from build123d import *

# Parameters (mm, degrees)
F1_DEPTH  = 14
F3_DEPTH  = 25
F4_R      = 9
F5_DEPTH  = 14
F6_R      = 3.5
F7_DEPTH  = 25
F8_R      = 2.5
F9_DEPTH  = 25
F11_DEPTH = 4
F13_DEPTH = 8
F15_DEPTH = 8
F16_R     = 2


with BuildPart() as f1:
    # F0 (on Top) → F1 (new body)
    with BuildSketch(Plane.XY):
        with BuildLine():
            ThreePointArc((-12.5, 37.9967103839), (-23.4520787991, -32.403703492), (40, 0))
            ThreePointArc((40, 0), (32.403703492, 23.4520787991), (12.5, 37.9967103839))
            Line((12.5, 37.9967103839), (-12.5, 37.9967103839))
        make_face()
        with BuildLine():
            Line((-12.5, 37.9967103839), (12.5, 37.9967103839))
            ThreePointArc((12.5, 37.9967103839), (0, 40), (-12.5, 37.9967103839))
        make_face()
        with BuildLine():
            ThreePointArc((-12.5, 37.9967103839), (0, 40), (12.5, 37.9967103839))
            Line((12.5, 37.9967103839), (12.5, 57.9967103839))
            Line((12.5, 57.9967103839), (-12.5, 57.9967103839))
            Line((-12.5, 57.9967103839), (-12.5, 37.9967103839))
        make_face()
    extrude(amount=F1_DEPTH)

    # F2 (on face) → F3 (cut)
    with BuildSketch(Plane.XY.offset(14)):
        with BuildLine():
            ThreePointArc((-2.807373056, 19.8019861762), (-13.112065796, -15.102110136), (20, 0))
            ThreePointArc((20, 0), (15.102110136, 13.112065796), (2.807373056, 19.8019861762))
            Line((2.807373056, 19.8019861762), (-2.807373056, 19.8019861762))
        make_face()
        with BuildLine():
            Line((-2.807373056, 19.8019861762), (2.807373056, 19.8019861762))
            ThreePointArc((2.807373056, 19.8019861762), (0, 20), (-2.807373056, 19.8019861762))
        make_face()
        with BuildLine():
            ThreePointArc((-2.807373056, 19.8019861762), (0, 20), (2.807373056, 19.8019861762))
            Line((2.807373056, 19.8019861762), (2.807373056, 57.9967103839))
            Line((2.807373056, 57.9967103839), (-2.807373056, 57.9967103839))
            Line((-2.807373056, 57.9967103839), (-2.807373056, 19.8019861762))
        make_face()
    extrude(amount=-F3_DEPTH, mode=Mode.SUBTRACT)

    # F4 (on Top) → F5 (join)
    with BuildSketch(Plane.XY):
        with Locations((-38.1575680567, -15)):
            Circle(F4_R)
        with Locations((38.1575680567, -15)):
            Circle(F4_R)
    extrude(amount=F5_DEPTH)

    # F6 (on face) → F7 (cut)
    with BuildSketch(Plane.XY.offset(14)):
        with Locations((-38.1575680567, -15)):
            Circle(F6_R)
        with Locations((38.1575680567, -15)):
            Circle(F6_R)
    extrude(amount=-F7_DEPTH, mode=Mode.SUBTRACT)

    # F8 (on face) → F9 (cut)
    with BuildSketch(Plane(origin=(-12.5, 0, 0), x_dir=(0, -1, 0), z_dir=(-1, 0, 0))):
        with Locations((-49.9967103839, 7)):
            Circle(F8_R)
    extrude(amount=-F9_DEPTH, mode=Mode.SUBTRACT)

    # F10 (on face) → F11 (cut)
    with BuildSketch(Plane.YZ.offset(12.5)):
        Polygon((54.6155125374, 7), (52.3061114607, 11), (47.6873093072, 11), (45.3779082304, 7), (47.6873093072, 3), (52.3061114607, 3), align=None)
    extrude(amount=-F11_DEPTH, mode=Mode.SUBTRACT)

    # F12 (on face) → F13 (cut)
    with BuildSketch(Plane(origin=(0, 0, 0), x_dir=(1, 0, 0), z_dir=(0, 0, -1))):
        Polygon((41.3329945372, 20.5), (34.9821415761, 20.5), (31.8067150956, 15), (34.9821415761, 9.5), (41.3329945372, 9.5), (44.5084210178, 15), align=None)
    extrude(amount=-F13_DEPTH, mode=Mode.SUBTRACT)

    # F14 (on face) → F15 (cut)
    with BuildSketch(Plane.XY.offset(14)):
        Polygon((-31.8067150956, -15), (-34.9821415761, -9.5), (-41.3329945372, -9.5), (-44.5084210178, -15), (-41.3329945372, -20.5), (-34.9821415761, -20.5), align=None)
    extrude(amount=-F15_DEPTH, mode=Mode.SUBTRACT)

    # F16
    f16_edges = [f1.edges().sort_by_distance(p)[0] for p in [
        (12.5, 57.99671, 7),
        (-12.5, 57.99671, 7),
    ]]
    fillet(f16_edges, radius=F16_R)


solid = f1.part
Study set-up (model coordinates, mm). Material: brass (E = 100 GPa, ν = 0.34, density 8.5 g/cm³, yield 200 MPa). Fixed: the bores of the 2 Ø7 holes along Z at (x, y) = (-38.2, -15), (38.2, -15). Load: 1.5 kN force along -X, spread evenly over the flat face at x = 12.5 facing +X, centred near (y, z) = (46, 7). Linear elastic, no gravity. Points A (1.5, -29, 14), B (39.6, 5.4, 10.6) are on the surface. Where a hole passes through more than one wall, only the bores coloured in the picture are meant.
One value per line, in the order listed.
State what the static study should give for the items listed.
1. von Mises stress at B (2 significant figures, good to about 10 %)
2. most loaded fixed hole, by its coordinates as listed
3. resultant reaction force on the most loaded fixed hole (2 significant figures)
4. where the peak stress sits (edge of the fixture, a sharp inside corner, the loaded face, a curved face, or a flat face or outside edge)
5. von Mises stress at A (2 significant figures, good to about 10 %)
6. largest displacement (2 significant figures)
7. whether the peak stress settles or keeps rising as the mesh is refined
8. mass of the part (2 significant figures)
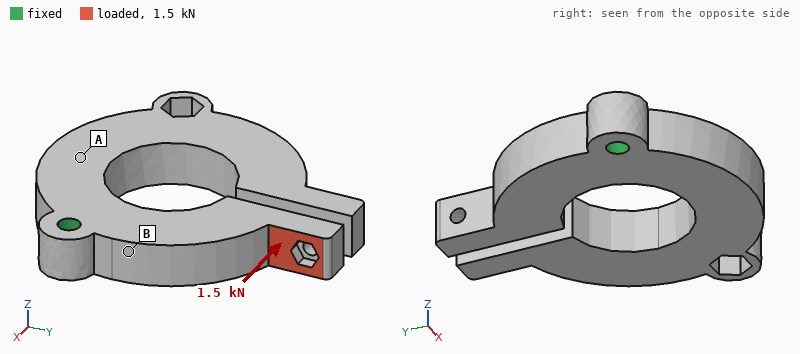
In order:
55 MPa
(38.2, -15)
3.0 kN
edge of the fixture
14 MPa
0.27 mm
keeps rising
490 g
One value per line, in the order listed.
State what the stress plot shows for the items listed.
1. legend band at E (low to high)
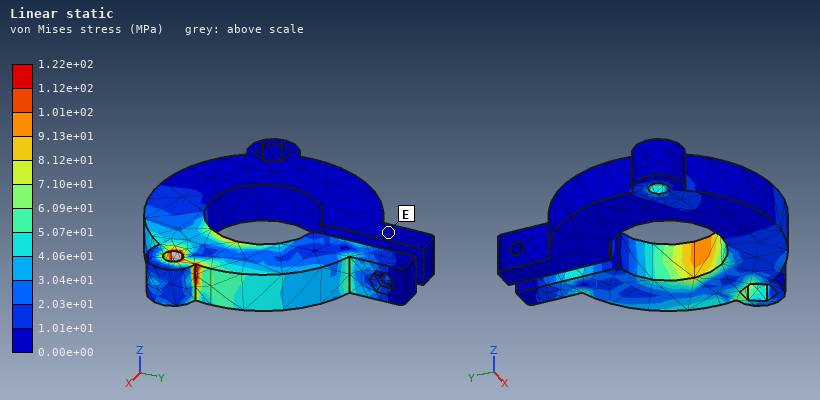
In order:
0.00e+00 to 1.01e+01 MPa
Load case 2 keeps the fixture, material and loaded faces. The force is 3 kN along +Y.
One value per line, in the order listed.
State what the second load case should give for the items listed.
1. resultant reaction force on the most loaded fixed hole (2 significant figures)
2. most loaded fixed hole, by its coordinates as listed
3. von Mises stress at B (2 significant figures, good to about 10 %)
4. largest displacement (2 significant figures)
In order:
2.5 kN
(38.2, -15)
34 MPa
0.14 mm
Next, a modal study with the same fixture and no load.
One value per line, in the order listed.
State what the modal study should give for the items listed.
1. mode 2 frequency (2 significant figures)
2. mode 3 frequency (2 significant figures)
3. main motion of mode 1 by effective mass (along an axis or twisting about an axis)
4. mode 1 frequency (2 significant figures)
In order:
1200 Hz
1800 Hz
along Z
1000 Hz
